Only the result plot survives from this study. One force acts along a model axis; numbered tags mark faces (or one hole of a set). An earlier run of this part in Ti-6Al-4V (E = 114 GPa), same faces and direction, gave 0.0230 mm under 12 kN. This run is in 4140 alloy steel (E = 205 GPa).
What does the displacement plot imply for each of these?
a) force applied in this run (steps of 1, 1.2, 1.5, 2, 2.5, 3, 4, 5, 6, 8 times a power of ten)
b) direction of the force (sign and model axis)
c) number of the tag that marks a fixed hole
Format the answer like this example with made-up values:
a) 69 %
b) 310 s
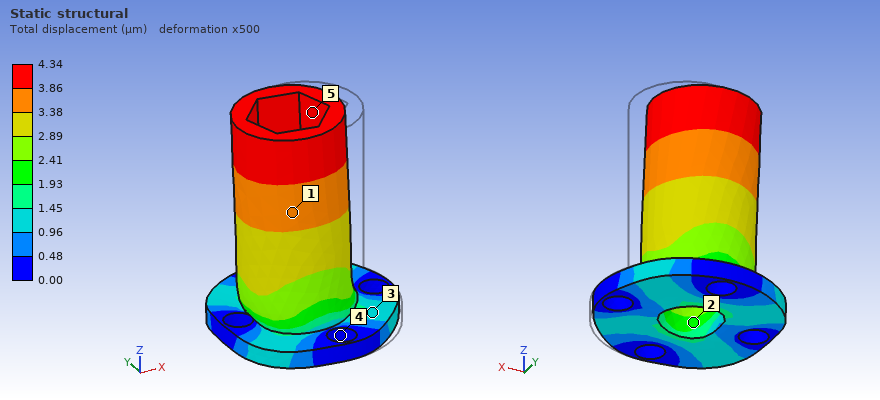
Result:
a) 4 kN
b) -X
c) 4
